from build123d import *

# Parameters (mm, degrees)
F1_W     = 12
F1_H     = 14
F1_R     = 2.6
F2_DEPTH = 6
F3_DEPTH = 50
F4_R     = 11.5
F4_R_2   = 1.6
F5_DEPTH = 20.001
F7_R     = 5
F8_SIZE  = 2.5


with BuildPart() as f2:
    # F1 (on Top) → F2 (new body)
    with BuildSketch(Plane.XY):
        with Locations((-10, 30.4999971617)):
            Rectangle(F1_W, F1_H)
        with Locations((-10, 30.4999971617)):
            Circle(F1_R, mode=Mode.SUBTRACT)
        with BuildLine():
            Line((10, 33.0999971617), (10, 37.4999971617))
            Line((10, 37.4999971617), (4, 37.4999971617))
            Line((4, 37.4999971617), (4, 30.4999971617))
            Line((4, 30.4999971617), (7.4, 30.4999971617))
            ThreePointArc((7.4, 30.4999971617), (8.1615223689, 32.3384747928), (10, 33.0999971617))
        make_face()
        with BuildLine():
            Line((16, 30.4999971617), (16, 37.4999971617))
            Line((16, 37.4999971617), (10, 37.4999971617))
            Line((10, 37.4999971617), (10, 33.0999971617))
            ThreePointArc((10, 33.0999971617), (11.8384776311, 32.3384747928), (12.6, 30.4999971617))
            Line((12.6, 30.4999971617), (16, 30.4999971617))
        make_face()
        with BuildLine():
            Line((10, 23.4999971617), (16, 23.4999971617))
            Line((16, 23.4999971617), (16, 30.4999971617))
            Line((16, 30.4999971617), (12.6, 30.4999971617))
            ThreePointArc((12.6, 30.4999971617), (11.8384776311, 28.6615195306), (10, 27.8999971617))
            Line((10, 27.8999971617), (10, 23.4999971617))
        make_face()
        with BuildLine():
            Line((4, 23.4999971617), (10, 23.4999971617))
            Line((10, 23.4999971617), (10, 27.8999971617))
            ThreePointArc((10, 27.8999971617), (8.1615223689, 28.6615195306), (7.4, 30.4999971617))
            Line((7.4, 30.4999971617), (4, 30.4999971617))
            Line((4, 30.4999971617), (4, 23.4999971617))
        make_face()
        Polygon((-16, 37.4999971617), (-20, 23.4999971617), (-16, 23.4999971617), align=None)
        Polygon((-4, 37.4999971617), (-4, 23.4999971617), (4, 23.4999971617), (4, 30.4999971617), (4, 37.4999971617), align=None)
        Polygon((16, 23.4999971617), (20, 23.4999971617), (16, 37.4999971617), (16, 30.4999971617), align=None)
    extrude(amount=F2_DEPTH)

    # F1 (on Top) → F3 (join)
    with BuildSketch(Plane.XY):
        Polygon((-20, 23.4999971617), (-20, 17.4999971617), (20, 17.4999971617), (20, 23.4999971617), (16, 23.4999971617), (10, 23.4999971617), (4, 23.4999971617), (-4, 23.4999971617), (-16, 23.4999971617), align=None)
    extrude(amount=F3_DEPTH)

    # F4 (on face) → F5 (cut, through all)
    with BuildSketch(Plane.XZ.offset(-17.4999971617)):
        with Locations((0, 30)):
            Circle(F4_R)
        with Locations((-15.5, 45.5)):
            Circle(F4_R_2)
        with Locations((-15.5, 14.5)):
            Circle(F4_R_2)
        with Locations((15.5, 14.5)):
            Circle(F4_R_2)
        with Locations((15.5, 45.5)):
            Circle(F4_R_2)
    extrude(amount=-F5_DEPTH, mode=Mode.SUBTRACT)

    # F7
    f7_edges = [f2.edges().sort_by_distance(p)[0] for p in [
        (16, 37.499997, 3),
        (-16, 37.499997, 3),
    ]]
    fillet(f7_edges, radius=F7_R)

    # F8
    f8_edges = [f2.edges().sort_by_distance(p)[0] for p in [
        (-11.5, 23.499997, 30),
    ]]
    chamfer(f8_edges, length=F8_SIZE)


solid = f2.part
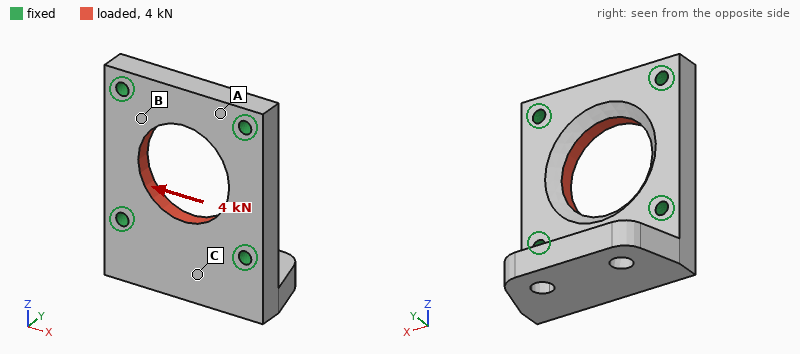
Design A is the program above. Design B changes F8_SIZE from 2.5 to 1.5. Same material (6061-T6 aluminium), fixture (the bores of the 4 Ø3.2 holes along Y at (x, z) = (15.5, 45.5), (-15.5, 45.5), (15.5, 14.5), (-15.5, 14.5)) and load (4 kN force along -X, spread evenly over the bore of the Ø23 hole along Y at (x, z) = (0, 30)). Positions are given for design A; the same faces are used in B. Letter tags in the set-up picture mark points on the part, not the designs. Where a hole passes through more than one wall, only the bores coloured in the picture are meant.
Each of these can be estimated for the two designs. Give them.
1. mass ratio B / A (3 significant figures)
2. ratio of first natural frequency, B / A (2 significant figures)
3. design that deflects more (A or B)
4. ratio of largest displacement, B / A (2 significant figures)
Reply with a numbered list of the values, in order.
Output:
1. 1.01
2. 1.0
3. A
4. 0.88
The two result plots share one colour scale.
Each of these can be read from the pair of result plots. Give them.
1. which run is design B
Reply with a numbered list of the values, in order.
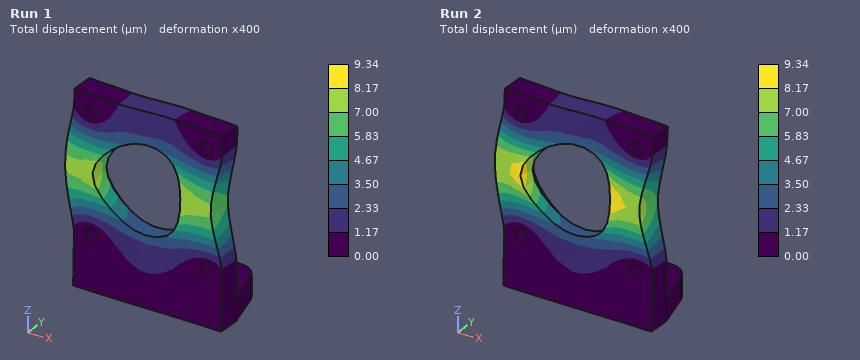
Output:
1. Run 1
